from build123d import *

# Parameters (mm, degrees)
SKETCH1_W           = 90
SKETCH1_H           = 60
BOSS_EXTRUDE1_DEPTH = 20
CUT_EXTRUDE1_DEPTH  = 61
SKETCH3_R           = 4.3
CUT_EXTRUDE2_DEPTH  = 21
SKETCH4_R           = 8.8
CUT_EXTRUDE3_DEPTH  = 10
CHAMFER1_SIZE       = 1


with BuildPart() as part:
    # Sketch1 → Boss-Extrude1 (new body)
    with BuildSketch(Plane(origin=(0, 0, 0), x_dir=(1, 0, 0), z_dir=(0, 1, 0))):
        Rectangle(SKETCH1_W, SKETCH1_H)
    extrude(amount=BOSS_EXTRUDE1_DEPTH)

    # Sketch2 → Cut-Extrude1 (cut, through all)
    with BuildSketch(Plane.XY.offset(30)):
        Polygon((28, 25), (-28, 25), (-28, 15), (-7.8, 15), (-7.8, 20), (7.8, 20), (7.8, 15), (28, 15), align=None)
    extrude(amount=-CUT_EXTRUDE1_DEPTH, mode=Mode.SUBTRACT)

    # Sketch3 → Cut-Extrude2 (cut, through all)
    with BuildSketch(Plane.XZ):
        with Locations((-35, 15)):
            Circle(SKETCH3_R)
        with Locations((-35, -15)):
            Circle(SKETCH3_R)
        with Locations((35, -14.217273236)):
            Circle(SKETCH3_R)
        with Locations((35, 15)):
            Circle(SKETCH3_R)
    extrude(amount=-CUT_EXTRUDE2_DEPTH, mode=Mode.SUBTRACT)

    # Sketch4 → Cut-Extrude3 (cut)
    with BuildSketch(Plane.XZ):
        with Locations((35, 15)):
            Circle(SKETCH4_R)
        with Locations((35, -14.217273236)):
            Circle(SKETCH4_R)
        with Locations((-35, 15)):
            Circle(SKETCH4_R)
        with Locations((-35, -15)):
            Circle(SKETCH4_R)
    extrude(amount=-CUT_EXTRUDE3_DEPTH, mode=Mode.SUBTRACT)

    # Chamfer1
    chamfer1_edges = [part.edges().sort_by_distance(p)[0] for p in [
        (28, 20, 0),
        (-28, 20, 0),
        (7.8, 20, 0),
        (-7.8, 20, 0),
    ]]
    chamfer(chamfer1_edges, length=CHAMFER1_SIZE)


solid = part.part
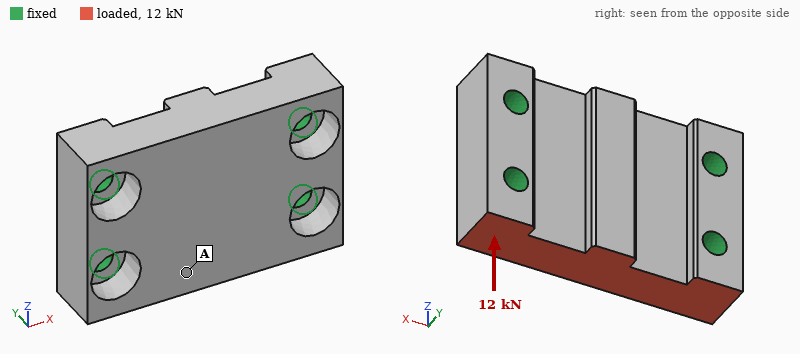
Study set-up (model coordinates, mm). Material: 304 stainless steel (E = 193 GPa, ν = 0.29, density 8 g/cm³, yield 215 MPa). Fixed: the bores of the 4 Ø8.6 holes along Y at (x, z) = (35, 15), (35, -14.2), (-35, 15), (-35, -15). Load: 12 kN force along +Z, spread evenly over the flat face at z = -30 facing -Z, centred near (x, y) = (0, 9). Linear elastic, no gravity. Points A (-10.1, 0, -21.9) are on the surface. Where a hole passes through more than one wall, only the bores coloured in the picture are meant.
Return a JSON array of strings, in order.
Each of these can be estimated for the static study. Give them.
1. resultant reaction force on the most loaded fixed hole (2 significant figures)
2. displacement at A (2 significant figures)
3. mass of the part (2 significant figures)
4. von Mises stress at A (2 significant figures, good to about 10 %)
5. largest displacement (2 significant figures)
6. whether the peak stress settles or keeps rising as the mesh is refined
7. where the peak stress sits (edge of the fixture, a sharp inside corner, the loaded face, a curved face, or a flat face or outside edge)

["4.1 kN", "3.4 µm", "670 g", "7.2 MPa", "4.7 µm", "keeps rising", "edge of the fixture"]
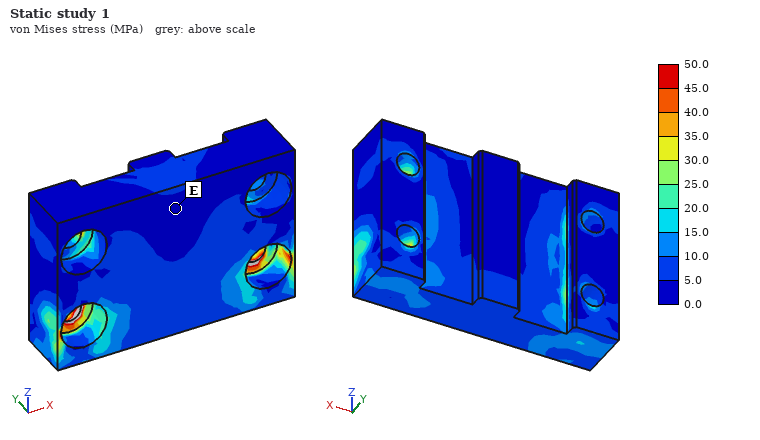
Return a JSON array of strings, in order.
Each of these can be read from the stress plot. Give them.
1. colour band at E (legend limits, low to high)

["0.0 to 5.0 MPa"]
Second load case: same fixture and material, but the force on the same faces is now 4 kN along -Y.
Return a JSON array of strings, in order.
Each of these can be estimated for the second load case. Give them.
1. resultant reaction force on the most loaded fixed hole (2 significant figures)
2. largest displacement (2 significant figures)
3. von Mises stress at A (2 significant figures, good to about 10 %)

["2.7 kN", "7.4 µm", "14 MPa"]
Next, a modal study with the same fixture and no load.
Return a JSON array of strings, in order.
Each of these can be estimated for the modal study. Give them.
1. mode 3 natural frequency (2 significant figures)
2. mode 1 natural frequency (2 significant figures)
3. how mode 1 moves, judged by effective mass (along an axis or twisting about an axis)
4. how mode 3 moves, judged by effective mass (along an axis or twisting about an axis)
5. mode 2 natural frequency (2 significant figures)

["14 kHz", "10 kHz", "along Y", "along Z", "11 kHz"]
